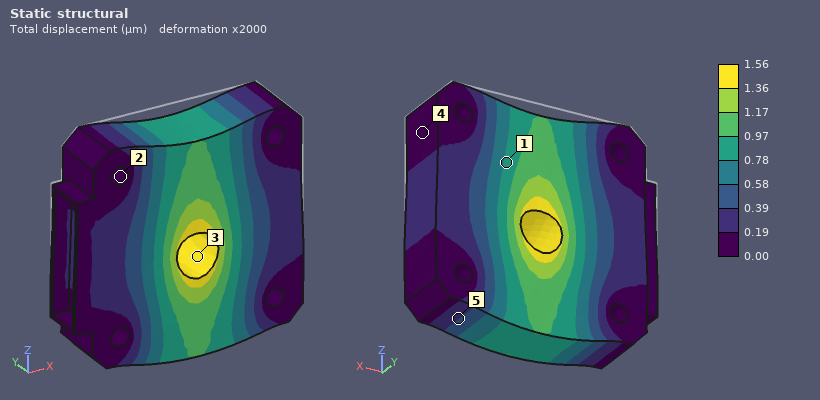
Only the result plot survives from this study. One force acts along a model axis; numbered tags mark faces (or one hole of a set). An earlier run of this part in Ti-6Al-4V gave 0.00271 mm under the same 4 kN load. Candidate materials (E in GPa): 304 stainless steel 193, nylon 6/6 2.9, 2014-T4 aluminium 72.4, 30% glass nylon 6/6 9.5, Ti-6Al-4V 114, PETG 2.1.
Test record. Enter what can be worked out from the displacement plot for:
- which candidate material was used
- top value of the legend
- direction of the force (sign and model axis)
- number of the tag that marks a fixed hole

304 stainless steel
1.56 µm
-Z
2
